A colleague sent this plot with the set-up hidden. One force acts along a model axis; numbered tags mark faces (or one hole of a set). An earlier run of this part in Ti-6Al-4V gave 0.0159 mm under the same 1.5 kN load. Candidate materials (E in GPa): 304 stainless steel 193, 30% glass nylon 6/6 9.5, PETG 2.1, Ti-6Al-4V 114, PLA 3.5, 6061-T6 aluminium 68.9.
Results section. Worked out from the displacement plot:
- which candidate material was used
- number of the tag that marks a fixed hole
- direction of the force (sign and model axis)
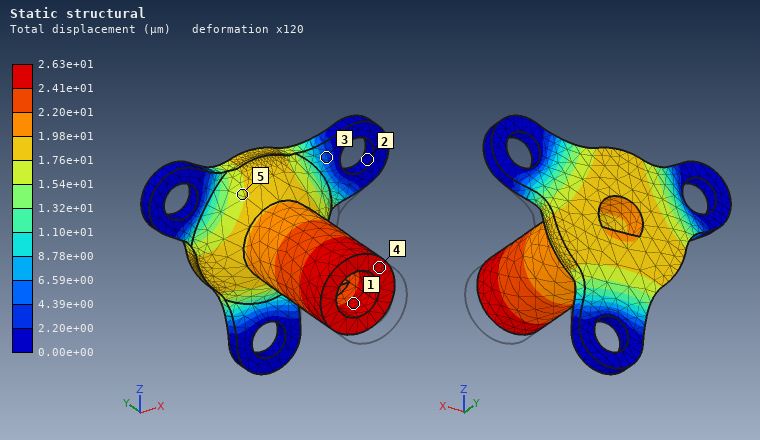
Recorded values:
6061-T6 aluminium
2
+Y
